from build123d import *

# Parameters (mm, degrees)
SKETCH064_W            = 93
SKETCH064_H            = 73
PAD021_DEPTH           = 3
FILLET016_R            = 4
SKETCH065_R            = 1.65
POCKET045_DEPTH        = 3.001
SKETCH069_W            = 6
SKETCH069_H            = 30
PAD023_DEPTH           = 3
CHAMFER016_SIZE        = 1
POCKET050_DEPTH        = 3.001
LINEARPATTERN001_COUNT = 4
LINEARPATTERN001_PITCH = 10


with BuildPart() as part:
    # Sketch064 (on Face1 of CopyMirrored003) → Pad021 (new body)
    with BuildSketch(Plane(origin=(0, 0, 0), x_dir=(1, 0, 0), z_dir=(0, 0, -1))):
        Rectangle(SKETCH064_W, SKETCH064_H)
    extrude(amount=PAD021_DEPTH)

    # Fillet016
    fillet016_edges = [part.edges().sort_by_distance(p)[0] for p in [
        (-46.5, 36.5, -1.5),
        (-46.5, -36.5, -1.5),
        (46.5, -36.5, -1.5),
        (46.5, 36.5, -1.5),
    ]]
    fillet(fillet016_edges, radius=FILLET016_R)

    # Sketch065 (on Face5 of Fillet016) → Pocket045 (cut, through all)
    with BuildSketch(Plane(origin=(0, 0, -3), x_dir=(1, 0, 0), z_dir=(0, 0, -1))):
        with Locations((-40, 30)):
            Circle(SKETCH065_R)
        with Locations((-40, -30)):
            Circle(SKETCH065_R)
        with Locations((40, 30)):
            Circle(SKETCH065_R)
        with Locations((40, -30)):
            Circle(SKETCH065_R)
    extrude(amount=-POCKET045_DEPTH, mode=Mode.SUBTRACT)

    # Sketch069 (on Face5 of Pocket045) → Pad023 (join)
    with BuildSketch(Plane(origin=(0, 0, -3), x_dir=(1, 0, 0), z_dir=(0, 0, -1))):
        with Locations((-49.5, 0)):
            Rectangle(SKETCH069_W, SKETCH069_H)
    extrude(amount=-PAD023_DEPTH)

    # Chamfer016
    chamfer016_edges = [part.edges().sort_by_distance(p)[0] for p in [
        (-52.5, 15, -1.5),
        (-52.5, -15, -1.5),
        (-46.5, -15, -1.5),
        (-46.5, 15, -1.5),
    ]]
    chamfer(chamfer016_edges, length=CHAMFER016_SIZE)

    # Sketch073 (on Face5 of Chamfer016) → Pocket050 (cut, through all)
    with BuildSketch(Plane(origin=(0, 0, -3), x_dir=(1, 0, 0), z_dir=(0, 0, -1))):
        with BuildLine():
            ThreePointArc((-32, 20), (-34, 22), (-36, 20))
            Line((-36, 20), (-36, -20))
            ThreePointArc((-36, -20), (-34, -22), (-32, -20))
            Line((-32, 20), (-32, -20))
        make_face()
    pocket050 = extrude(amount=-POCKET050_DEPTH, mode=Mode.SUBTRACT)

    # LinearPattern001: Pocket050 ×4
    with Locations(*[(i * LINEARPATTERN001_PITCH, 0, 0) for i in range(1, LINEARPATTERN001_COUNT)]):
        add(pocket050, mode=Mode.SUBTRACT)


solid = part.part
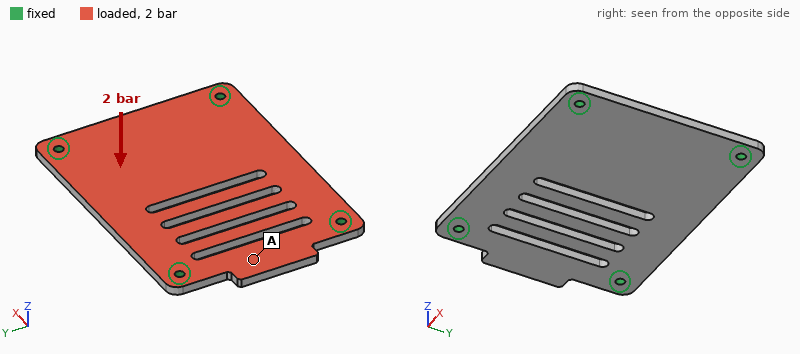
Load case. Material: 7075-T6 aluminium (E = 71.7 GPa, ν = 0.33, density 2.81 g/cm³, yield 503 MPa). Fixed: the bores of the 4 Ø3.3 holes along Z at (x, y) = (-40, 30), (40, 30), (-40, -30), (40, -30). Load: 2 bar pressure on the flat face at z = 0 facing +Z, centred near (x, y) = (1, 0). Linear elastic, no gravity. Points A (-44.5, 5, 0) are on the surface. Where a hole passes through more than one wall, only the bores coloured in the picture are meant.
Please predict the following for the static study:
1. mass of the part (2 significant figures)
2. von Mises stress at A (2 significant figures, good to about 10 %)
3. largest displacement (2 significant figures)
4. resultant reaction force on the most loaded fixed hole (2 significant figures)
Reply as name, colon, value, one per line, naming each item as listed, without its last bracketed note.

mass of the part: 53 g
von Mises stress at A: 17 MPa
largest displacement: 0.35 mm
resultant reaction force on the most loaded fixed hole: 320 N
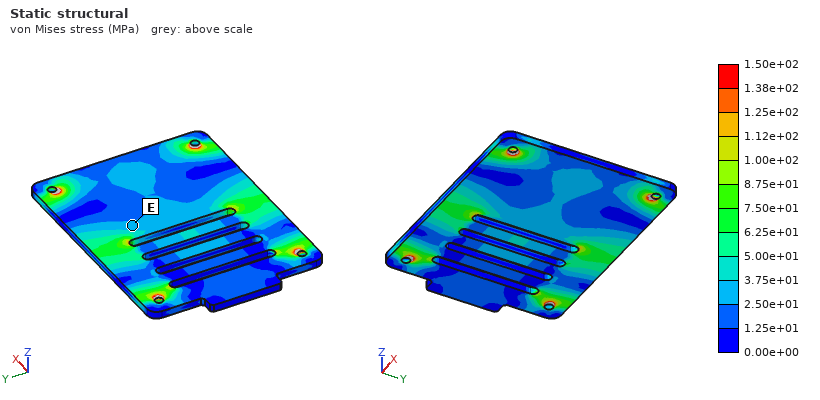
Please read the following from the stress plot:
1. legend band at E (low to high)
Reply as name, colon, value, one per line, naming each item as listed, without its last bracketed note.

legend band at E: 2.50e+01 to 3.75e+01 MPa
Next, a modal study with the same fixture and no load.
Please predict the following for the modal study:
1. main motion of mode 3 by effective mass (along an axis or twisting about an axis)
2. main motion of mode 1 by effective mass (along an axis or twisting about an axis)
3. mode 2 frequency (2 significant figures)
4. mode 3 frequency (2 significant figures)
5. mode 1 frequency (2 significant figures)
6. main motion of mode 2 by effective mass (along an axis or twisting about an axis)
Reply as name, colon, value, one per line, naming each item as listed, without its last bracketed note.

main motion of mode 3 by effective mass: twisting about Y
main motion of mode 1 by effective mass: along Z
mode 2 frequency: 2800 Hz
mode 3 frequency: 3600 Hz
mode 1 frequency: 1700 Hz
main motion of mode 2 by effective mass: twisting about X
